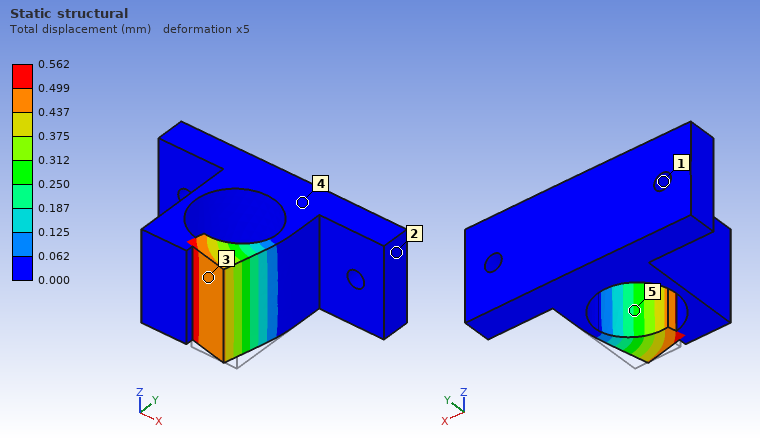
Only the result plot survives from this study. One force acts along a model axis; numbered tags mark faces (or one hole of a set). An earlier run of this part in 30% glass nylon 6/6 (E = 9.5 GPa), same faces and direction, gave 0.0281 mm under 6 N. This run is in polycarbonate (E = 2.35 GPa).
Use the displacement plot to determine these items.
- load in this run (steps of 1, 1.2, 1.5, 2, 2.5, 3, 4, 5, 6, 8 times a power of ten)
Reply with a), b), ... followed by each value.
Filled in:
a) 30 N
